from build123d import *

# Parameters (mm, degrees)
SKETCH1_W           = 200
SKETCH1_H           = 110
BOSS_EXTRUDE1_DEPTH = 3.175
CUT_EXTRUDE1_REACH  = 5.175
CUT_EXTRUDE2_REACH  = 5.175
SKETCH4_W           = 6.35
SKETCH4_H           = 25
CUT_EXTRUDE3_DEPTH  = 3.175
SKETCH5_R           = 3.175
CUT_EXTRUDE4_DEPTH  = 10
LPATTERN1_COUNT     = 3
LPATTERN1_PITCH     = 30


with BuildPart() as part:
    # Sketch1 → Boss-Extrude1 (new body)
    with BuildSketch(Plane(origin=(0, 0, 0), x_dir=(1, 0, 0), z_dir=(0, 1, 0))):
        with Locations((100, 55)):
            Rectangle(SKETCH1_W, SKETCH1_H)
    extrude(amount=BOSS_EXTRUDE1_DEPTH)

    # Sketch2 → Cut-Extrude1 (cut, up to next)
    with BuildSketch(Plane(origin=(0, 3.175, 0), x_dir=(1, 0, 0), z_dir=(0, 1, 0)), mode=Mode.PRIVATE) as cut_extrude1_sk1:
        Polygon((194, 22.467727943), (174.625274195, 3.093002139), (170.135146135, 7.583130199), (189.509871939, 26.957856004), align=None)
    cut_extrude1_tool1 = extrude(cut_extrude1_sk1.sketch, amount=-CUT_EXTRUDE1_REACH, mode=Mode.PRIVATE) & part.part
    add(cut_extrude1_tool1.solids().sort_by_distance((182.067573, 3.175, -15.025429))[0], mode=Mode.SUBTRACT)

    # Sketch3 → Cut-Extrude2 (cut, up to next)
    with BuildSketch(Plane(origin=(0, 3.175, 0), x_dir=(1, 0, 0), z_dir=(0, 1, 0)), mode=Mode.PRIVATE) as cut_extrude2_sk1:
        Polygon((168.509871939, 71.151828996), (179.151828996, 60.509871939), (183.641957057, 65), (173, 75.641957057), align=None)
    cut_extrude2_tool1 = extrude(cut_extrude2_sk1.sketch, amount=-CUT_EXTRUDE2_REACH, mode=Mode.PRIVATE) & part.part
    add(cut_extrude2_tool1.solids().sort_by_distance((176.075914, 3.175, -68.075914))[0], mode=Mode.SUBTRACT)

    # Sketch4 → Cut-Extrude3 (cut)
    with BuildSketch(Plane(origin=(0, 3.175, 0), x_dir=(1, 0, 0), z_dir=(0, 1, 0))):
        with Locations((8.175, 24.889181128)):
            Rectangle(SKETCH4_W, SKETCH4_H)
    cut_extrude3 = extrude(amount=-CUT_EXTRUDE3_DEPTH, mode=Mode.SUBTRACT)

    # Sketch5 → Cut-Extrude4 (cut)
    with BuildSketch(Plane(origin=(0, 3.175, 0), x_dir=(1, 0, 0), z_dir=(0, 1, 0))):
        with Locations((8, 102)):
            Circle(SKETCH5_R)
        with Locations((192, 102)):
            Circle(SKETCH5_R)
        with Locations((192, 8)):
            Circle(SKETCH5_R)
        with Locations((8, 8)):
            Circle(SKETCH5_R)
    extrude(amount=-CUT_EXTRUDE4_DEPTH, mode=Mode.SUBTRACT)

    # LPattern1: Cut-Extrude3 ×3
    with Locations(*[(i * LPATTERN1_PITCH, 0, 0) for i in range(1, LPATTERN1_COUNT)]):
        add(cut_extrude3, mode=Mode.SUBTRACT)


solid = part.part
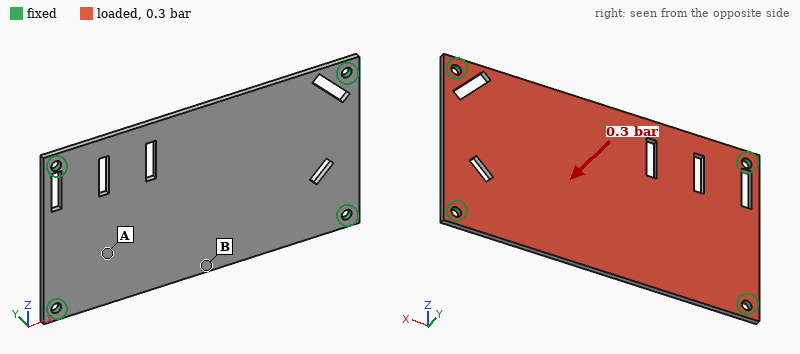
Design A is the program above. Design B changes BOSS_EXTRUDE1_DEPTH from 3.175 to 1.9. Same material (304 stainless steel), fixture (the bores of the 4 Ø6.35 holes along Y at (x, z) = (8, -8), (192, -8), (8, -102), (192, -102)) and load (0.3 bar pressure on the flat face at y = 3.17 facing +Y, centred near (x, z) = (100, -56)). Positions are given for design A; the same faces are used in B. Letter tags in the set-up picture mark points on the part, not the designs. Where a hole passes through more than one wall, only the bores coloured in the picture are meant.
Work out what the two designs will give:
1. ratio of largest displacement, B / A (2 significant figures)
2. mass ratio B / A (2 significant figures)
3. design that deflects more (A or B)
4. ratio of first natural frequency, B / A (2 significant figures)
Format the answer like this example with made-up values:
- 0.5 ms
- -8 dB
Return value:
- 4.5
- 0.60
- B
- 0.61
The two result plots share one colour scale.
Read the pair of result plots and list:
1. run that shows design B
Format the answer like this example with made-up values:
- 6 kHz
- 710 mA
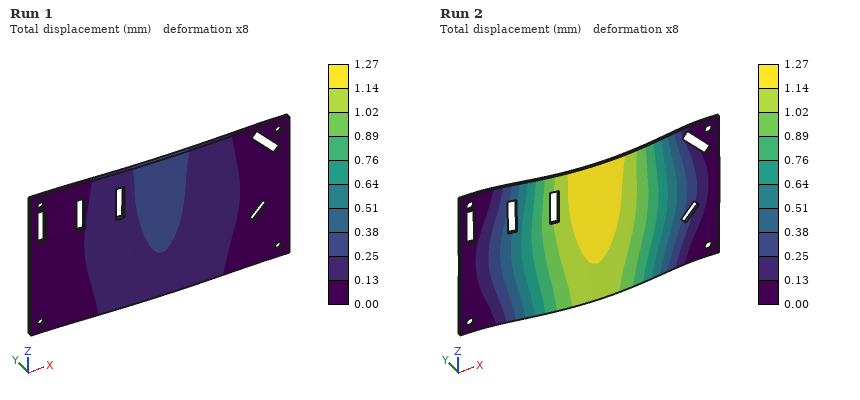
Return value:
- Run 2
